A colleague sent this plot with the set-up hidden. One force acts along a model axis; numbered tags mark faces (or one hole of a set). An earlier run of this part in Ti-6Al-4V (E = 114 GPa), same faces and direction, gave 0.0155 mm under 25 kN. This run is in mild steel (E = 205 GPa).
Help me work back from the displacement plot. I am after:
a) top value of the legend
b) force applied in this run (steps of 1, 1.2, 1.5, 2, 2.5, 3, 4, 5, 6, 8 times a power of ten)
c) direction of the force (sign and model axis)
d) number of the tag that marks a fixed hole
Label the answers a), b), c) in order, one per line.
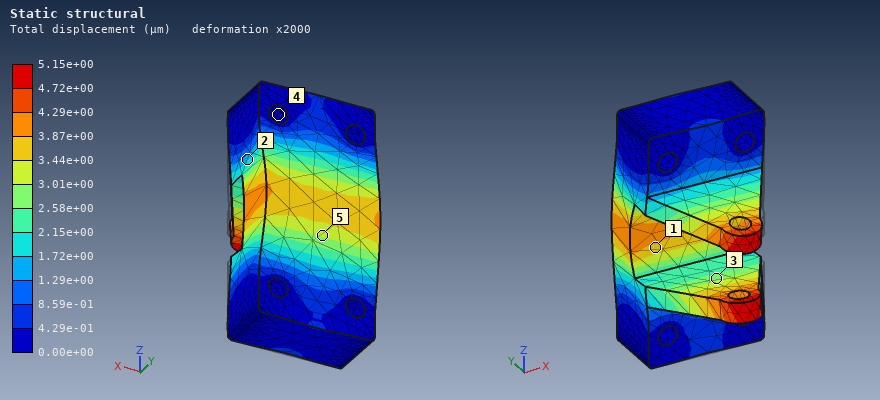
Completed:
a) 5.15e+00 µm
b) 15 kN
c) +Y
d) 4
